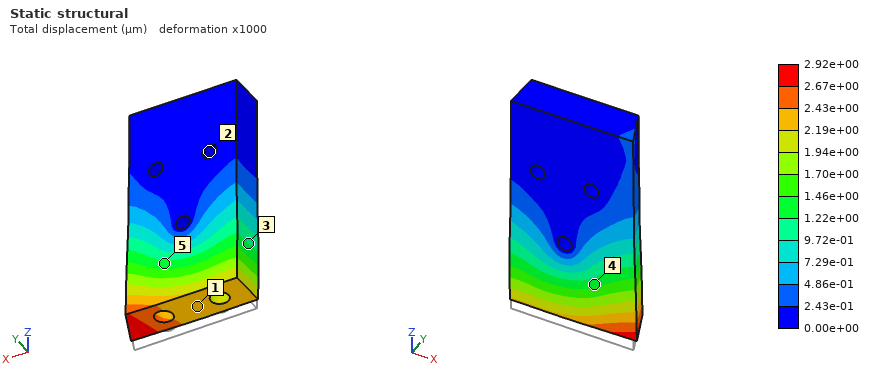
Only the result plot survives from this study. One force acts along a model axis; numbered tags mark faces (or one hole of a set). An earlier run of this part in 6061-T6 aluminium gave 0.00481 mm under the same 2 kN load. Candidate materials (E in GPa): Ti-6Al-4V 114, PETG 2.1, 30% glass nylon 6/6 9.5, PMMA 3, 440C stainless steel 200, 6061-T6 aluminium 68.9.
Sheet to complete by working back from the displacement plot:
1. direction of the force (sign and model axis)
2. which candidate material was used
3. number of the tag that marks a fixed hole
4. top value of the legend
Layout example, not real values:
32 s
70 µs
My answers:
+Z
Ti-6Al-4V
2
2.92e+00 µm
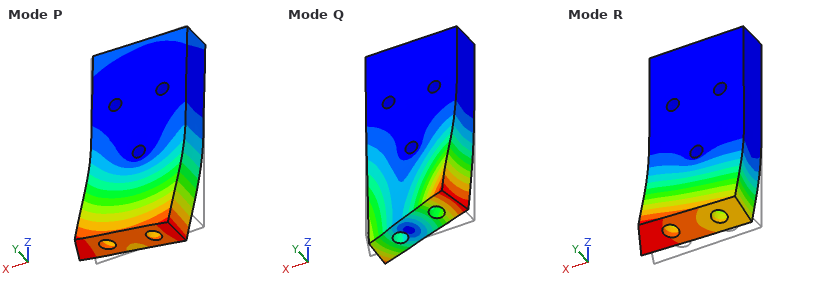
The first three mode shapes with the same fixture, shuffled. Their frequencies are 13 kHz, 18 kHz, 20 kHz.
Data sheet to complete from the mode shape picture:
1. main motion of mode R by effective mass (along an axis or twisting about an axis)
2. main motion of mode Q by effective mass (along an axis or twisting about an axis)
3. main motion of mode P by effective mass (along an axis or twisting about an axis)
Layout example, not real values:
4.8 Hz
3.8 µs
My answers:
along Y
twisting about Z
along X
